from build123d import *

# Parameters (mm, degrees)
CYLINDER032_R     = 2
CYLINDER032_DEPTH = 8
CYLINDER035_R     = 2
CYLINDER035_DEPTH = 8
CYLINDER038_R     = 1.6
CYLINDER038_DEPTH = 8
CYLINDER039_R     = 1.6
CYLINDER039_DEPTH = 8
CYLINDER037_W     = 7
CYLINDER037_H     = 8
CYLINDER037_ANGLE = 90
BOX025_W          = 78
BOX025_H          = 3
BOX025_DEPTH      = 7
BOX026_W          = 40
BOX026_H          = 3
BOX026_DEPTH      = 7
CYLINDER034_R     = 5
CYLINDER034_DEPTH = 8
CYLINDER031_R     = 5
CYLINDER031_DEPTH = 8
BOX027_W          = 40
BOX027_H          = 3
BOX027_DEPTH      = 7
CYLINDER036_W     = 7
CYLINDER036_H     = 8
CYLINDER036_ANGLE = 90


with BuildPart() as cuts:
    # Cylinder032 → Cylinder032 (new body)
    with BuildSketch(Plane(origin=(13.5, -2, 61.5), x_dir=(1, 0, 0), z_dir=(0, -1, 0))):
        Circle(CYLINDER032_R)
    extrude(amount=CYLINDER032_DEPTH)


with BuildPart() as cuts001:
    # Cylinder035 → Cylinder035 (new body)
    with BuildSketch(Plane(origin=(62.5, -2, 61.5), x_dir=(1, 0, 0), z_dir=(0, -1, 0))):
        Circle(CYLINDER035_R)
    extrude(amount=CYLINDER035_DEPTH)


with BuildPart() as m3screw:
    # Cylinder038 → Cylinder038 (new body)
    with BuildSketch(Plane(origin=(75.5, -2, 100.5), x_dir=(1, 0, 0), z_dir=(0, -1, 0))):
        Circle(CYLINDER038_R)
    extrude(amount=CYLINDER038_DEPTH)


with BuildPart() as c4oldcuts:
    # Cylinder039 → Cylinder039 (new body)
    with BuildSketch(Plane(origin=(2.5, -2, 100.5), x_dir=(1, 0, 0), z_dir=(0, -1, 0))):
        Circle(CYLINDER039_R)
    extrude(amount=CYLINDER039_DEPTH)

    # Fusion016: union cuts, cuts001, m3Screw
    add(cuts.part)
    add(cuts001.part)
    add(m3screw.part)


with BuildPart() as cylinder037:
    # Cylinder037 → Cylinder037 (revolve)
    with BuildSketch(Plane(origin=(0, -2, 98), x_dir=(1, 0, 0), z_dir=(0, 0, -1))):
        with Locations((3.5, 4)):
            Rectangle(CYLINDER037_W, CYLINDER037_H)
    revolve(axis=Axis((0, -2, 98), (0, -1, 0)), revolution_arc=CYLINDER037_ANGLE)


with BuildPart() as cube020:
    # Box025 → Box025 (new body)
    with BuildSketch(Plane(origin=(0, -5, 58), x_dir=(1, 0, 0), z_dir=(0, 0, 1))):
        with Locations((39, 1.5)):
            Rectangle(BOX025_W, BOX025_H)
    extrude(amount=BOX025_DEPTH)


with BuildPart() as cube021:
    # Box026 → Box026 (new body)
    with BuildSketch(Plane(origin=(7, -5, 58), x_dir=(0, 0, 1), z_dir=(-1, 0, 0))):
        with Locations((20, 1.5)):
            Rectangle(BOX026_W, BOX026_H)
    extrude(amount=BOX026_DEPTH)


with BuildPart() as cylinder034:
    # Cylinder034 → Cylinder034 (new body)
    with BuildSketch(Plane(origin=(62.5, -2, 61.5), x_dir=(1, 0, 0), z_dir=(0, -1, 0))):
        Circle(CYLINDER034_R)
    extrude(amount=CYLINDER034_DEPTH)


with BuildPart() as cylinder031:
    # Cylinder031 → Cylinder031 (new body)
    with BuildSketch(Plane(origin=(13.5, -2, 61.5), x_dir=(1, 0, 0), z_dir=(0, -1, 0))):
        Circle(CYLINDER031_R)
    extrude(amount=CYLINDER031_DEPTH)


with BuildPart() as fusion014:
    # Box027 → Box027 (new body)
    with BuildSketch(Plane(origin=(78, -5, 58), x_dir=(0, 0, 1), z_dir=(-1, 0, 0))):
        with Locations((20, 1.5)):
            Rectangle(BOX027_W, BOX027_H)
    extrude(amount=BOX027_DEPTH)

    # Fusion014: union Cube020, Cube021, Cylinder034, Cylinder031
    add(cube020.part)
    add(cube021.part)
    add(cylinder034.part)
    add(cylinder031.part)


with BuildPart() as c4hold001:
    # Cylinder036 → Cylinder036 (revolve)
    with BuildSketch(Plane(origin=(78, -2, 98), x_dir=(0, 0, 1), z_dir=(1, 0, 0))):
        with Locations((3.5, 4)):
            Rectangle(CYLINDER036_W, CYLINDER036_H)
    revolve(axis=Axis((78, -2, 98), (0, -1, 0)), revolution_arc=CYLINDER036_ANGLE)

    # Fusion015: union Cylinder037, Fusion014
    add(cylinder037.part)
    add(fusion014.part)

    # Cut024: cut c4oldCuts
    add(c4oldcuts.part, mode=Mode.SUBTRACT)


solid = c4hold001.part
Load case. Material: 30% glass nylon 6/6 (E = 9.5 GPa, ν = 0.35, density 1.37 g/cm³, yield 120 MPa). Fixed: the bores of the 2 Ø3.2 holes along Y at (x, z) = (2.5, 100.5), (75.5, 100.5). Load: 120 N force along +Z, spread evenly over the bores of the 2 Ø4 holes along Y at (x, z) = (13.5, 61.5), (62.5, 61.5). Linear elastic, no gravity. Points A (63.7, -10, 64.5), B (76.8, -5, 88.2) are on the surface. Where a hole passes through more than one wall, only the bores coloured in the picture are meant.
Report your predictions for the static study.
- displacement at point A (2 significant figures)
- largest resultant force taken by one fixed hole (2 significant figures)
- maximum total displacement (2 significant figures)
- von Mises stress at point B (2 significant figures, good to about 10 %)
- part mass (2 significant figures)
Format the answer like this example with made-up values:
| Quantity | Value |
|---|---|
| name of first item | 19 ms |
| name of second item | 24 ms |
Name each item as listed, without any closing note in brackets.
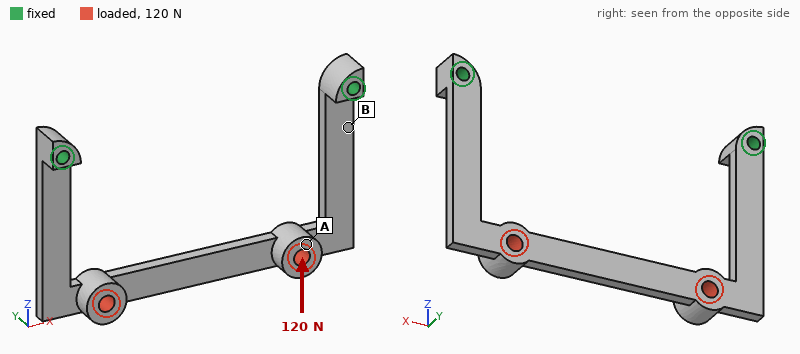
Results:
| Quantity | Value |
|---|---|
| displacement at point A | 0.67 mm |
| largest resultant force taken by one fixed hole | 64 N |
| maximum total displacement | 0.98 mm |
| von Mises stress at point B | 17 MPa |
| part mass | 5.7 g |
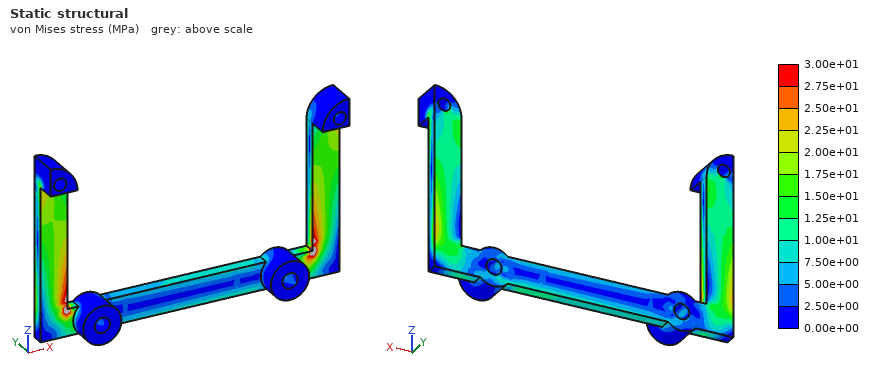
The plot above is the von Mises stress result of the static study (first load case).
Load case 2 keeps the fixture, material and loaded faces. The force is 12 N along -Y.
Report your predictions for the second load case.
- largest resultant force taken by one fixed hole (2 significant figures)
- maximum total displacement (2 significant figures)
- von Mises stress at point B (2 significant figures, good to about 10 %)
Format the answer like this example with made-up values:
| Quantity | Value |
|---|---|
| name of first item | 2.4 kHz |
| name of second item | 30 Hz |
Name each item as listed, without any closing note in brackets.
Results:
| Quantity | Value |
|---|---|
| largest resultant force taken by one fixed hole | 6.2 N |
| maximum total displacement | 0.95 mm |
| von Mises stress at point B | 15 MPa |
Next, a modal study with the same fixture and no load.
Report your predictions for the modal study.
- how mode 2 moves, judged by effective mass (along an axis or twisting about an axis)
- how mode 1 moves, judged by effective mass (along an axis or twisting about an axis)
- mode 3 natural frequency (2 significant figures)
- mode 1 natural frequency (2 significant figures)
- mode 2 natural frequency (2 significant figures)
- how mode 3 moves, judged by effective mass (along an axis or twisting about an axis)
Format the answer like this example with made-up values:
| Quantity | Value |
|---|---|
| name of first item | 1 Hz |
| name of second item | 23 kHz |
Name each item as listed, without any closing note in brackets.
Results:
| Quantity | Value |
|---|---|
| how mode 2 moves, judged by effective mass | twisting about Z |
| how mode 1 moves, judged by effective mass | along Y |
| mode 3 natural frequency | 1200 Hz |
| mode 1 natural frequency | 330 Hz |
| mode 2 natural frequency | 700 Hz |
| how mode 3 moves, judged by effective mass | along X |
